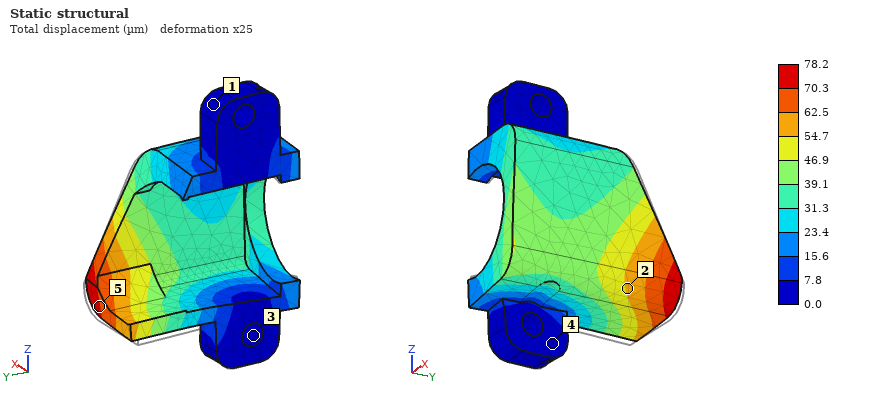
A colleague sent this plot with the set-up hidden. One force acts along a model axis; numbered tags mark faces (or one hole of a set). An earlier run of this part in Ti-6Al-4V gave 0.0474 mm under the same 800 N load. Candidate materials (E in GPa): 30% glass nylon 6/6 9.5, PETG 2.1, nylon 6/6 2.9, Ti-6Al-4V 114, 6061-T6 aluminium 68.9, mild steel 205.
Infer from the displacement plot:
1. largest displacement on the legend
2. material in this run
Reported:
78.2 µm
6061-T6 aluminium
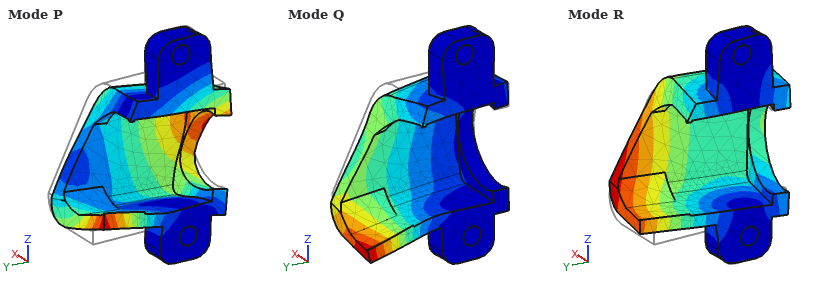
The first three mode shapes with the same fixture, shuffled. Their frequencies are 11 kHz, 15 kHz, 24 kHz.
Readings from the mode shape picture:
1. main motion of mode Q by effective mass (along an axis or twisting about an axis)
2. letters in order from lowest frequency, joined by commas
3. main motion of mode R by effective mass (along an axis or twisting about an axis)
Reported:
along Z
R, Q, P
along Y
